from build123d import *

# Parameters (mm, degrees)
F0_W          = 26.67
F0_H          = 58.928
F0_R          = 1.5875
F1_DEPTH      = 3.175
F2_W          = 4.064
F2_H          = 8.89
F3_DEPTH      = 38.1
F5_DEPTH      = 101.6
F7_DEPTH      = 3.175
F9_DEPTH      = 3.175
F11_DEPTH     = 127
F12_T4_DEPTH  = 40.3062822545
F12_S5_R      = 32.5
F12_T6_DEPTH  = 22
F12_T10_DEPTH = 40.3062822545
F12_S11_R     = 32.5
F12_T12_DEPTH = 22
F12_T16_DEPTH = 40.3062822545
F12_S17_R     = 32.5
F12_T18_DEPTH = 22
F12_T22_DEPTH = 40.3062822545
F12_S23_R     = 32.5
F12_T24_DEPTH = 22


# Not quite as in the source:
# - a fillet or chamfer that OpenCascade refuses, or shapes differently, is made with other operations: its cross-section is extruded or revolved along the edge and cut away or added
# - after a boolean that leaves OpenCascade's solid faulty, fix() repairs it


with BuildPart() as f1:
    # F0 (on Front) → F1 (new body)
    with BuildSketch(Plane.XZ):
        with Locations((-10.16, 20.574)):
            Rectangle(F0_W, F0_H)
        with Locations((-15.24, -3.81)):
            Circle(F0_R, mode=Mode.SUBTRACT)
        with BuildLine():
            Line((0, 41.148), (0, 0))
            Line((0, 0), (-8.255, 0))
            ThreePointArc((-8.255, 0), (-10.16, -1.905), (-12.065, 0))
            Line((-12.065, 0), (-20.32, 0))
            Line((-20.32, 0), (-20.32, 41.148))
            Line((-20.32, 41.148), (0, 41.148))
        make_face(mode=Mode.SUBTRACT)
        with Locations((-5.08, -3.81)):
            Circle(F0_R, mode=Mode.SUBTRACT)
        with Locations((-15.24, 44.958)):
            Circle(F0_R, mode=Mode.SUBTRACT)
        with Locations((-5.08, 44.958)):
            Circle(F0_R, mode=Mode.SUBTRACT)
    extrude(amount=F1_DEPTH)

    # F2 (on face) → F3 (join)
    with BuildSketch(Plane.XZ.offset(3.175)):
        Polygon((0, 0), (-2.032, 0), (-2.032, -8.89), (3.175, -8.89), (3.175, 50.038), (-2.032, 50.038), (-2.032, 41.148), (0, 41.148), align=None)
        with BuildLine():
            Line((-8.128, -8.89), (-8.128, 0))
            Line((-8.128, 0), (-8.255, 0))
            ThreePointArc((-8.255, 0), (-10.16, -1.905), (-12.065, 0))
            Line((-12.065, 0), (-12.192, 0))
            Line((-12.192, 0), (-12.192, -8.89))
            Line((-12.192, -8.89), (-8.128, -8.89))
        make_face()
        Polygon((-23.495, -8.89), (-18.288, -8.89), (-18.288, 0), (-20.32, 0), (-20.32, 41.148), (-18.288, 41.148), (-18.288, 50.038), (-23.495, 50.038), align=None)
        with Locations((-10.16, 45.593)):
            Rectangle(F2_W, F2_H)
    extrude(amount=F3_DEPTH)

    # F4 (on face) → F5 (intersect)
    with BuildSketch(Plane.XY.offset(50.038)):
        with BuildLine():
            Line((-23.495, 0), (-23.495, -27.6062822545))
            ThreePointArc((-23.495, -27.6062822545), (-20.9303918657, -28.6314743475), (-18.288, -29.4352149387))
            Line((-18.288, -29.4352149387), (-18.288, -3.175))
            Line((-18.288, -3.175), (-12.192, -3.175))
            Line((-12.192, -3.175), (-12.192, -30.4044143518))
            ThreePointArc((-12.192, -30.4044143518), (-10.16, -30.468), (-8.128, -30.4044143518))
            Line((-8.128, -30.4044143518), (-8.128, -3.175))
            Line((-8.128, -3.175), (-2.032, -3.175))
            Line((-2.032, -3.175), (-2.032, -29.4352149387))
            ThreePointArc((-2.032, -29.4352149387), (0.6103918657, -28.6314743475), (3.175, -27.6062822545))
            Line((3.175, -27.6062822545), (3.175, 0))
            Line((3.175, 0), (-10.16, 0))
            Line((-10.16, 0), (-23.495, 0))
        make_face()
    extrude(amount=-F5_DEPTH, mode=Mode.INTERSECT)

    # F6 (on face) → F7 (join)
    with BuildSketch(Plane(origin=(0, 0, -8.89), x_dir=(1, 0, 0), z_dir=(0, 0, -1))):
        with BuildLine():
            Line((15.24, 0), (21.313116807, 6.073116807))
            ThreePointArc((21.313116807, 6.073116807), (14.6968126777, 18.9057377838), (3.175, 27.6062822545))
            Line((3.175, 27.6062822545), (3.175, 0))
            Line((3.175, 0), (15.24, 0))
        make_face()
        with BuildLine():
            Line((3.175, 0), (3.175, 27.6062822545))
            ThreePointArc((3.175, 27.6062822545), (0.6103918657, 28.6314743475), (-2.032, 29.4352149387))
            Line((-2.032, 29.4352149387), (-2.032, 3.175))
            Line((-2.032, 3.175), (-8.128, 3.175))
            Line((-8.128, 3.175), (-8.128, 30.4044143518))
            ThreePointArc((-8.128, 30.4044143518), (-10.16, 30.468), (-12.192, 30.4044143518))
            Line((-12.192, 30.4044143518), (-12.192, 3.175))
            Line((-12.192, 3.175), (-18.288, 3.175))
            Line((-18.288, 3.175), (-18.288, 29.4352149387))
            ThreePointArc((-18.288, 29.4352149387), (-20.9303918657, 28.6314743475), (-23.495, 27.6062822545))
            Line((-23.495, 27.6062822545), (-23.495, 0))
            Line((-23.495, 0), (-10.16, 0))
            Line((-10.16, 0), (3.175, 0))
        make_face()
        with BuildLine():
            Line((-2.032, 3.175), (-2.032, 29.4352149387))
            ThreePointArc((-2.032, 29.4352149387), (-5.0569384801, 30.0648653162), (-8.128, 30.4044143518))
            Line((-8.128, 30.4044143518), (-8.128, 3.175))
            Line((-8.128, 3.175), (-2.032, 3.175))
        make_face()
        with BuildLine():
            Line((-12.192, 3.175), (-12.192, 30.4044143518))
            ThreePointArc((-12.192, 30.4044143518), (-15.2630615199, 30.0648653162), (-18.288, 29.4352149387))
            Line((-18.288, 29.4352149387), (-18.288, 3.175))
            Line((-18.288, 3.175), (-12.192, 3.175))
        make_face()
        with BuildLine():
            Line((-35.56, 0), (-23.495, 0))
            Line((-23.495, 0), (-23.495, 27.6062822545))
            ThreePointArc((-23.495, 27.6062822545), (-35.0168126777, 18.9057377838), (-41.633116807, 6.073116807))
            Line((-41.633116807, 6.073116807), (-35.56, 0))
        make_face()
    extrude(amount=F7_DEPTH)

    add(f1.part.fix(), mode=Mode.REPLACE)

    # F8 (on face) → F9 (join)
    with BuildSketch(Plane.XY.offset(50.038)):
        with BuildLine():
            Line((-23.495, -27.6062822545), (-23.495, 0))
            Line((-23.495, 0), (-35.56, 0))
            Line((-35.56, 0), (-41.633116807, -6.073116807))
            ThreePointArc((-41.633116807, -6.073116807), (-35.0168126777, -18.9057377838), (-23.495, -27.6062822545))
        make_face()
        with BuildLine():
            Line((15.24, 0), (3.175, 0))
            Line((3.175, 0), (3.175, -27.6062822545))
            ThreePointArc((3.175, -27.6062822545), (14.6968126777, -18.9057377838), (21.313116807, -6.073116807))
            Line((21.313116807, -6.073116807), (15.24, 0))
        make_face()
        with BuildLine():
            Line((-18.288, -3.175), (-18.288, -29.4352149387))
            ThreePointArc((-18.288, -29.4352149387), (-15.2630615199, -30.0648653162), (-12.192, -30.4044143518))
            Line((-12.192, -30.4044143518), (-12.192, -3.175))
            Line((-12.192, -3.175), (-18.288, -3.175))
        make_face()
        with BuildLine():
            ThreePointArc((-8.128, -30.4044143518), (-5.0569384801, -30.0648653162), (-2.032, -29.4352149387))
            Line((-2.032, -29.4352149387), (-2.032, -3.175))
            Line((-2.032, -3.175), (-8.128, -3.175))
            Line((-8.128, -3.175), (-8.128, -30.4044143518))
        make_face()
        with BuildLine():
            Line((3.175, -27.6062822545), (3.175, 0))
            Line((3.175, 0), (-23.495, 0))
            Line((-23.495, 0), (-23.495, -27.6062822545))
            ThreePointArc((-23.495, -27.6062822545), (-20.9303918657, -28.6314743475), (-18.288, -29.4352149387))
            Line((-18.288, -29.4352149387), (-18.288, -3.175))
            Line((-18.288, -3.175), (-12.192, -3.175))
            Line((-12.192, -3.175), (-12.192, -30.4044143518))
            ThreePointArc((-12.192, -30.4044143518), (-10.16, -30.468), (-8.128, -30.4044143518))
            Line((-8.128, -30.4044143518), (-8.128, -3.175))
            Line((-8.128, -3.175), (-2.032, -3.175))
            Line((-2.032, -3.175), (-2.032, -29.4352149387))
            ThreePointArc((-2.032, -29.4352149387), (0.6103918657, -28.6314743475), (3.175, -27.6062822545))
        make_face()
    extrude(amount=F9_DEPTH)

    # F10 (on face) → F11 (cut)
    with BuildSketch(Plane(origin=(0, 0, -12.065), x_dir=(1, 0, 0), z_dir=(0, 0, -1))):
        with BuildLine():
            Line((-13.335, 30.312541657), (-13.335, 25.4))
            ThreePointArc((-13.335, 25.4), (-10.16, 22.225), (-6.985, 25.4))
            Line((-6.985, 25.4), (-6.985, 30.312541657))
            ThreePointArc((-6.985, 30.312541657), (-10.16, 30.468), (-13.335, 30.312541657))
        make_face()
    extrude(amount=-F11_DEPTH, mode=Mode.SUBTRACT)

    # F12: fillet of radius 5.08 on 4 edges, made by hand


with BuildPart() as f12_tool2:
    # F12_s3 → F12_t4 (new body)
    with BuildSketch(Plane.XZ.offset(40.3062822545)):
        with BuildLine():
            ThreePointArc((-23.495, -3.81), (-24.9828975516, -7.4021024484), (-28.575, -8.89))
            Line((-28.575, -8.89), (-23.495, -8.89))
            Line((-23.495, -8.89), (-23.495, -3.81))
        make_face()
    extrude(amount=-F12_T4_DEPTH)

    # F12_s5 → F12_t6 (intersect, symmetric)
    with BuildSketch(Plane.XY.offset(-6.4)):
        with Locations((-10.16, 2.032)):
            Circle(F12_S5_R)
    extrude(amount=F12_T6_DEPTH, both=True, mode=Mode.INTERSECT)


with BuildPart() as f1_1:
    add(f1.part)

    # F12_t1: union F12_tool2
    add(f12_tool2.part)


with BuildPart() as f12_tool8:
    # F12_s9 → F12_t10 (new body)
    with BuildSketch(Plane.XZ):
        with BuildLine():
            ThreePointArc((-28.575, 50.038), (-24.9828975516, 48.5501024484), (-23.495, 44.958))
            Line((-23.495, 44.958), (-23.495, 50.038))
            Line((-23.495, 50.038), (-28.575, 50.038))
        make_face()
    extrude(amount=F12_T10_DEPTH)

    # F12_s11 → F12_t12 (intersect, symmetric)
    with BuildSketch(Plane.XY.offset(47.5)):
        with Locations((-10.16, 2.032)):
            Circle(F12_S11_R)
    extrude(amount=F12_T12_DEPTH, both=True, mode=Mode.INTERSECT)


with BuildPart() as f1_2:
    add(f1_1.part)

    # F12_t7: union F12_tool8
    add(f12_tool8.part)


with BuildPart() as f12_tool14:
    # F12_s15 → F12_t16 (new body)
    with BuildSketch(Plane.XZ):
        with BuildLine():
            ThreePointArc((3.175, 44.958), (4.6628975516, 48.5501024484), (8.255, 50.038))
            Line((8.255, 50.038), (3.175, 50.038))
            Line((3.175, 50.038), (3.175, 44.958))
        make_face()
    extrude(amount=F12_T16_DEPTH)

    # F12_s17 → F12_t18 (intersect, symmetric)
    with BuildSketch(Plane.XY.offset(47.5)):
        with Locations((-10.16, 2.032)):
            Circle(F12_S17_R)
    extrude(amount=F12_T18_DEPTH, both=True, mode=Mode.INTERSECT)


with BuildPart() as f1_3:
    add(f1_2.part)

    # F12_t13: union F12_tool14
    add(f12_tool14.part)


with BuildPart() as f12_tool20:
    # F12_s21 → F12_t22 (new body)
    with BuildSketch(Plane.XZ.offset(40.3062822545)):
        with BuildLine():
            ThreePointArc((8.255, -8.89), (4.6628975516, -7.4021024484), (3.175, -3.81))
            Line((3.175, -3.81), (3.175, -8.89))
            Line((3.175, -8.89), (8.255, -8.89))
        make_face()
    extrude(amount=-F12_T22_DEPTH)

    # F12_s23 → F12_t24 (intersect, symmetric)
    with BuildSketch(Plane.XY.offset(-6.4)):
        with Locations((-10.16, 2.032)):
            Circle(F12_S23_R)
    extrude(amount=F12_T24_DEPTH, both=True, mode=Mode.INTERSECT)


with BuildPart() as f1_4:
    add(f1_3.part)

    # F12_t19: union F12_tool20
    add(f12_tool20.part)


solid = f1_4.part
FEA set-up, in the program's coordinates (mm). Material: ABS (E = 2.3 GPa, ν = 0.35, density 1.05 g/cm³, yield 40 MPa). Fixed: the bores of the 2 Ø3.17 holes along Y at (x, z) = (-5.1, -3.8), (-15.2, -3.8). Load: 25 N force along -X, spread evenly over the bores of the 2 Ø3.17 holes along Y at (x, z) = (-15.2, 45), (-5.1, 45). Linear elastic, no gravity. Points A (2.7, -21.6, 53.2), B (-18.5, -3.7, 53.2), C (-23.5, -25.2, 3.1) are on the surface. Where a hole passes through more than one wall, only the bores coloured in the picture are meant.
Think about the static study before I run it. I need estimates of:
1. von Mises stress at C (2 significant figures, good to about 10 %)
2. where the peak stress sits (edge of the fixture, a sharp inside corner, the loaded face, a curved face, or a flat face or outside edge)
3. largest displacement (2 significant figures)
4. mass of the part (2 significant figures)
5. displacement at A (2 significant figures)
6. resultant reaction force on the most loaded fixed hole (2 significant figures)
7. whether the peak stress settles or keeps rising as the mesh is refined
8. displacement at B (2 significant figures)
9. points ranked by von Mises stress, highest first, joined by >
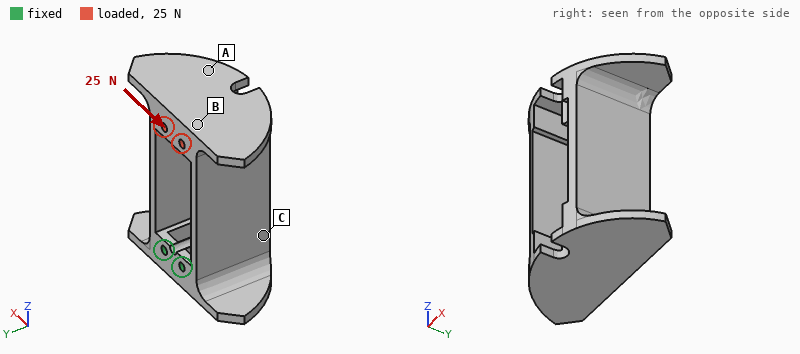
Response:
3.2 MPa
edge of the fixture
1.1 mm
26 g
0.89 mm
82 N
keeps rising
1.0 mm
C > B > A
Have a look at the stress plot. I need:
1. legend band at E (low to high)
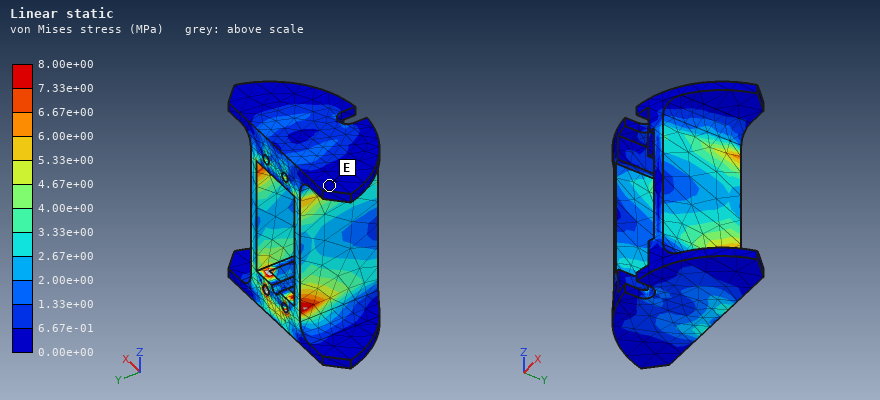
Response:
0.00e+00 to 6.67e-01 MPa
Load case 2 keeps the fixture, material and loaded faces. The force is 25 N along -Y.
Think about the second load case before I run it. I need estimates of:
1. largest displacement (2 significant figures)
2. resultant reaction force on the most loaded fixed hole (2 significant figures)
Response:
0.98 mm
13 N
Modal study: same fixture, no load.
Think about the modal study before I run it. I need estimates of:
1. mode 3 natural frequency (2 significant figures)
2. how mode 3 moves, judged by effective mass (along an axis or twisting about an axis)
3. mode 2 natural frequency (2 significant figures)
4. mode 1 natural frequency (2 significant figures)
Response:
620 Hz
twisting about Z
240 Hz
240 Hz
